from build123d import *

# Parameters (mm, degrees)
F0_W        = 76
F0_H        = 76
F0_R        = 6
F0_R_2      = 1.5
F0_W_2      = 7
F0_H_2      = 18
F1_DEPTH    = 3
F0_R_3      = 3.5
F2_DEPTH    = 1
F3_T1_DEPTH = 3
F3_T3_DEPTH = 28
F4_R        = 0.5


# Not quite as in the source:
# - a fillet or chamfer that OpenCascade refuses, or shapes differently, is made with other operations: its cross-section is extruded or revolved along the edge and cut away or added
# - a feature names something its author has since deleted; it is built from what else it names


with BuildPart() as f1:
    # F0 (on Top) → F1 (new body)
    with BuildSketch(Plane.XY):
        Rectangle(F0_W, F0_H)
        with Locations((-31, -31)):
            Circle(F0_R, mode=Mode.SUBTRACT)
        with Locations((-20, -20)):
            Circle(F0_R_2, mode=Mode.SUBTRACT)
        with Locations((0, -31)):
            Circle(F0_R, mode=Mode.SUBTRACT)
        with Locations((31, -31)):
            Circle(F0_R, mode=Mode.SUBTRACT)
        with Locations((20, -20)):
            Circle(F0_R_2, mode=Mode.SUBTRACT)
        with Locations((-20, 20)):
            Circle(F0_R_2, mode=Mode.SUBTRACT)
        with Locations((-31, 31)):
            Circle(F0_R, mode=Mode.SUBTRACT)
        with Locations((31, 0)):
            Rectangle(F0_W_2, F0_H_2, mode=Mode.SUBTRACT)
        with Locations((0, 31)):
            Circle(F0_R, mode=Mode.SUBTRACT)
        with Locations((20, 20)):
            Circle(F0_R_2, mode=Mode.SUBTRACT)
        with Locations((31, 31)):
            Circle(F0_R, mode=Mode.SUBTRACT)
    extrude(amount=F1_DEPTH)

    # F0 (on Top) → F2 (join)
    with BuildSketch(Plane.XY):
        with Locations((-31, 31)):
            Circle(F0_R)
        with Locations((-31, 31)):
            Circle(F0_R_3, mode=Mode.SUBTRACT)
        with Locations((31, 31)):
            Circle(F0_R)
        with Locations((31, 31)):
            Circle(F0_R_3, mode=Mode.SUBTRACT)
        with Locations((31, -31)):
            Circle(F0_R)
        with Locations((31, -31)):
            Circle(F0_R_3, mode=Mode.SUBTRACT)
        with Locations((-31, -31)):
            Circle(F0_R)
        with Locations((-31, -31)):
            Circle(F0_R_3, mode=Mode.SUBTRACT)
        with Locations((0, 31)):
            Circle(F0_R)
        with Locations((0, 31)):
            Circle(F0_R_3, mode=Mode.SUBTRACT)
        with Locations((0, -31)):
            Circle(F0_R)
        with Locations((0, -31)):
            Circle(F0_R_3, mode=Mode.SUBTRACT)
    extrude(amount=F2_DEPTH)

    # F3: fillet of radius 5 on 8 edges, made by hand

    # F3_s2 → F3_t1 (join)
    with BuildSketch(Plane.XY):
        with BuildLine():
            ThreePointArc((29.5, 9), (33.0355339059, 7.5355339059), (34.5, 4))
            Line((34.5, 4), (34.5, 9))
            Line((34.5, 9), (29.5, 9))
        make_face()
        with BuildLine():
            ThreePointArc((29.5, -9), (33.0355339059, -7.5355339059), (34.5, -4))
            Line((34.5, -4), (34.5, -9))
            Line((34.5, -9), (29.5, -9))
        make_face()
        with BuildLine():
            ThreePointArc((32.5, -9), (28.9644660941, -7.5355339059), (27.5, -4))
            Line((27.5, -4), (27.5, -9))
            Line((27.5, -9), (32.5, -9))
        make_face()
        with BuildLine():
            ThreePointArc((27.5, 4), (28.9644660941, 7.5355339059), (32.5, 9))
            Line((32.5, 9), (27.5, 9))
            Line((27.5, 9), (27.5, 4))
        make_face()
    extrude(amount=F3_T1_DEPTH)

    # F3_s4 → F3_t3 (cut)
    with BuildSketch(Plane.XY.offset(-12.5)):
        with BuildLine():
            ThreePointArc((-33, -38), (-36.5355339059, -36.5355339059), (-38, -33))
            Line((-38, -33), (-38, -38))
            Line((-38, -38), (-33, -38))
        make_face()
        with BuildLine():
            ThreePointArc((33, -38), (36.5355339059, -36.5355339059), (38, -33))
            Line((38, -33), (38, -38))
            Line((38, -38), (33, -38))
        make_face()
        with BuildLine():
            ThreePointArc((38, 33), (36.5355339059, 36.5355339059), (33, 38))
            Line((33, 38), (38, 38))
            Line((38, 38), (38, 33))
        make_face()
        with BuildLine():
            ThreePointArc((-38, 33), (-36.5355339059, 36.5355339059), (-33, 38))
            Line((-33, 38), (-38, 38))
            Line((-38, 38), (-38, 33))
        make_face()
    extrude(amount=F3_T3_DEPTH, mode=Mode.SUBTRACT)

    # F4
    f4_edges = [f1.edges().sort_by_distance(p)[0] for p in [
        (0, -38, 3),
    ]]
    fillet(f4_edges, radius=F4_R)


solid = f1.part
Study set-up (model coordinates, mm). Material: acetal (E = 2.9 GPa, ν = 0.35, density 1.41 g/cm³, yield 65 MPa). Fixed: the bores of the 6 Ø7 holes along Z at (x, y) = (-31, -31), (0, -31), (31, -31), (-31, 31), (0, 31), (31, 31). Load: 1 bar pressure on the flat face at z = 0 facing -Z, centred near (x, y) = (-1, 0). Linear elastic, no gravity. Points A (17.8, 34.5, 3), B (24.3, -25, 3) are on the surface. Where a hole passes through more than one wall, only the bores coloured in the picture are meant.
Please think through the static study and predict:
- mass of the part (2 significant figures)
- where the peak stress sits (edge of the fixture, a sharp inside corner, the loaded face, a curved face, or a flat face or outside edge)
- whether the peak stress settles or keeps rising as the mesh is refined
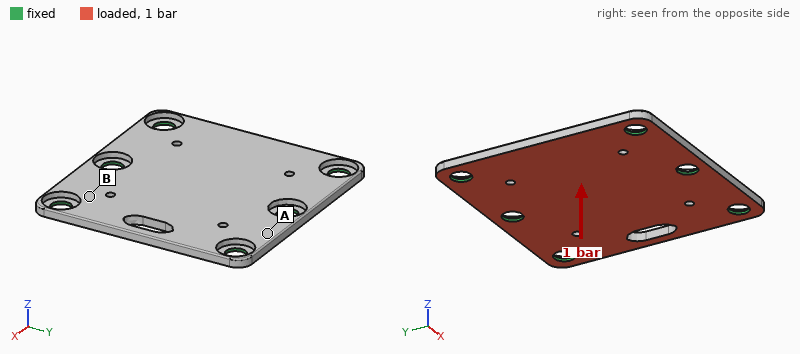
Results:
22 g
edge of the fixture
keeps rising
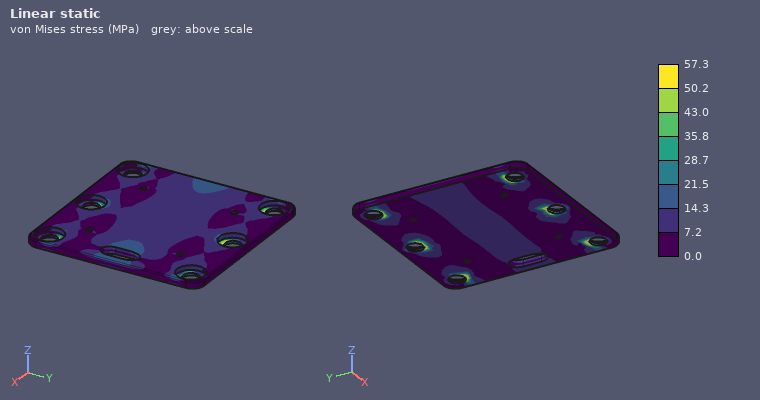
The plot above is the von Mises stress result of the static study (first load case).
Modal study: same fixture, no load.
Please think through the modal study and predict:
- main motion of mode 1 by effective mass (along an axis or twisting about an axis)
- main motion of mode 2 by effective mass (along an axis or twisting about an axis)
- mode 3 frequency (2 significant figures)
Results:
along Z
twisting about Y
1800 Hz
